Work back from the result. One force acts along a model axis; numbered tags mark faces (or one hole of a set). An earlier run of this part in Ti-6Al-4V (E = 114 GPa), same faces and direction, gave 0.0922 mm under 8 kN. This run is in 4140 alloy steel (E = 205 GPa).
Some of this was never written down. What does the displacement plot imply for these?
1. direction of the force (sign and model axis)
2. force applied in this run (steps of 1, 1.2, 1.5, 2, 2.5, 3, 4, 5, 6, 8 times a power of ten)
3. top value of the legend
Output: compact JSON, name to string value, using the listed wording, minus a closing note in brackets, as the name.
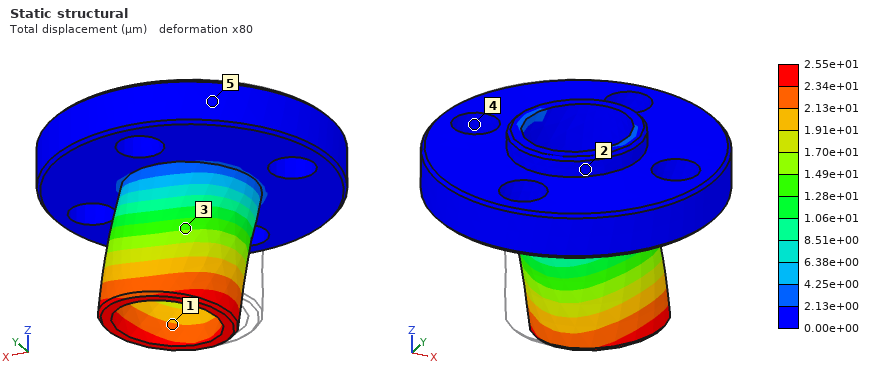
{"direction of the force": "+X", "force applied in this run": "4 kN", "top value of the legend": "2.55e+01 µm"}
